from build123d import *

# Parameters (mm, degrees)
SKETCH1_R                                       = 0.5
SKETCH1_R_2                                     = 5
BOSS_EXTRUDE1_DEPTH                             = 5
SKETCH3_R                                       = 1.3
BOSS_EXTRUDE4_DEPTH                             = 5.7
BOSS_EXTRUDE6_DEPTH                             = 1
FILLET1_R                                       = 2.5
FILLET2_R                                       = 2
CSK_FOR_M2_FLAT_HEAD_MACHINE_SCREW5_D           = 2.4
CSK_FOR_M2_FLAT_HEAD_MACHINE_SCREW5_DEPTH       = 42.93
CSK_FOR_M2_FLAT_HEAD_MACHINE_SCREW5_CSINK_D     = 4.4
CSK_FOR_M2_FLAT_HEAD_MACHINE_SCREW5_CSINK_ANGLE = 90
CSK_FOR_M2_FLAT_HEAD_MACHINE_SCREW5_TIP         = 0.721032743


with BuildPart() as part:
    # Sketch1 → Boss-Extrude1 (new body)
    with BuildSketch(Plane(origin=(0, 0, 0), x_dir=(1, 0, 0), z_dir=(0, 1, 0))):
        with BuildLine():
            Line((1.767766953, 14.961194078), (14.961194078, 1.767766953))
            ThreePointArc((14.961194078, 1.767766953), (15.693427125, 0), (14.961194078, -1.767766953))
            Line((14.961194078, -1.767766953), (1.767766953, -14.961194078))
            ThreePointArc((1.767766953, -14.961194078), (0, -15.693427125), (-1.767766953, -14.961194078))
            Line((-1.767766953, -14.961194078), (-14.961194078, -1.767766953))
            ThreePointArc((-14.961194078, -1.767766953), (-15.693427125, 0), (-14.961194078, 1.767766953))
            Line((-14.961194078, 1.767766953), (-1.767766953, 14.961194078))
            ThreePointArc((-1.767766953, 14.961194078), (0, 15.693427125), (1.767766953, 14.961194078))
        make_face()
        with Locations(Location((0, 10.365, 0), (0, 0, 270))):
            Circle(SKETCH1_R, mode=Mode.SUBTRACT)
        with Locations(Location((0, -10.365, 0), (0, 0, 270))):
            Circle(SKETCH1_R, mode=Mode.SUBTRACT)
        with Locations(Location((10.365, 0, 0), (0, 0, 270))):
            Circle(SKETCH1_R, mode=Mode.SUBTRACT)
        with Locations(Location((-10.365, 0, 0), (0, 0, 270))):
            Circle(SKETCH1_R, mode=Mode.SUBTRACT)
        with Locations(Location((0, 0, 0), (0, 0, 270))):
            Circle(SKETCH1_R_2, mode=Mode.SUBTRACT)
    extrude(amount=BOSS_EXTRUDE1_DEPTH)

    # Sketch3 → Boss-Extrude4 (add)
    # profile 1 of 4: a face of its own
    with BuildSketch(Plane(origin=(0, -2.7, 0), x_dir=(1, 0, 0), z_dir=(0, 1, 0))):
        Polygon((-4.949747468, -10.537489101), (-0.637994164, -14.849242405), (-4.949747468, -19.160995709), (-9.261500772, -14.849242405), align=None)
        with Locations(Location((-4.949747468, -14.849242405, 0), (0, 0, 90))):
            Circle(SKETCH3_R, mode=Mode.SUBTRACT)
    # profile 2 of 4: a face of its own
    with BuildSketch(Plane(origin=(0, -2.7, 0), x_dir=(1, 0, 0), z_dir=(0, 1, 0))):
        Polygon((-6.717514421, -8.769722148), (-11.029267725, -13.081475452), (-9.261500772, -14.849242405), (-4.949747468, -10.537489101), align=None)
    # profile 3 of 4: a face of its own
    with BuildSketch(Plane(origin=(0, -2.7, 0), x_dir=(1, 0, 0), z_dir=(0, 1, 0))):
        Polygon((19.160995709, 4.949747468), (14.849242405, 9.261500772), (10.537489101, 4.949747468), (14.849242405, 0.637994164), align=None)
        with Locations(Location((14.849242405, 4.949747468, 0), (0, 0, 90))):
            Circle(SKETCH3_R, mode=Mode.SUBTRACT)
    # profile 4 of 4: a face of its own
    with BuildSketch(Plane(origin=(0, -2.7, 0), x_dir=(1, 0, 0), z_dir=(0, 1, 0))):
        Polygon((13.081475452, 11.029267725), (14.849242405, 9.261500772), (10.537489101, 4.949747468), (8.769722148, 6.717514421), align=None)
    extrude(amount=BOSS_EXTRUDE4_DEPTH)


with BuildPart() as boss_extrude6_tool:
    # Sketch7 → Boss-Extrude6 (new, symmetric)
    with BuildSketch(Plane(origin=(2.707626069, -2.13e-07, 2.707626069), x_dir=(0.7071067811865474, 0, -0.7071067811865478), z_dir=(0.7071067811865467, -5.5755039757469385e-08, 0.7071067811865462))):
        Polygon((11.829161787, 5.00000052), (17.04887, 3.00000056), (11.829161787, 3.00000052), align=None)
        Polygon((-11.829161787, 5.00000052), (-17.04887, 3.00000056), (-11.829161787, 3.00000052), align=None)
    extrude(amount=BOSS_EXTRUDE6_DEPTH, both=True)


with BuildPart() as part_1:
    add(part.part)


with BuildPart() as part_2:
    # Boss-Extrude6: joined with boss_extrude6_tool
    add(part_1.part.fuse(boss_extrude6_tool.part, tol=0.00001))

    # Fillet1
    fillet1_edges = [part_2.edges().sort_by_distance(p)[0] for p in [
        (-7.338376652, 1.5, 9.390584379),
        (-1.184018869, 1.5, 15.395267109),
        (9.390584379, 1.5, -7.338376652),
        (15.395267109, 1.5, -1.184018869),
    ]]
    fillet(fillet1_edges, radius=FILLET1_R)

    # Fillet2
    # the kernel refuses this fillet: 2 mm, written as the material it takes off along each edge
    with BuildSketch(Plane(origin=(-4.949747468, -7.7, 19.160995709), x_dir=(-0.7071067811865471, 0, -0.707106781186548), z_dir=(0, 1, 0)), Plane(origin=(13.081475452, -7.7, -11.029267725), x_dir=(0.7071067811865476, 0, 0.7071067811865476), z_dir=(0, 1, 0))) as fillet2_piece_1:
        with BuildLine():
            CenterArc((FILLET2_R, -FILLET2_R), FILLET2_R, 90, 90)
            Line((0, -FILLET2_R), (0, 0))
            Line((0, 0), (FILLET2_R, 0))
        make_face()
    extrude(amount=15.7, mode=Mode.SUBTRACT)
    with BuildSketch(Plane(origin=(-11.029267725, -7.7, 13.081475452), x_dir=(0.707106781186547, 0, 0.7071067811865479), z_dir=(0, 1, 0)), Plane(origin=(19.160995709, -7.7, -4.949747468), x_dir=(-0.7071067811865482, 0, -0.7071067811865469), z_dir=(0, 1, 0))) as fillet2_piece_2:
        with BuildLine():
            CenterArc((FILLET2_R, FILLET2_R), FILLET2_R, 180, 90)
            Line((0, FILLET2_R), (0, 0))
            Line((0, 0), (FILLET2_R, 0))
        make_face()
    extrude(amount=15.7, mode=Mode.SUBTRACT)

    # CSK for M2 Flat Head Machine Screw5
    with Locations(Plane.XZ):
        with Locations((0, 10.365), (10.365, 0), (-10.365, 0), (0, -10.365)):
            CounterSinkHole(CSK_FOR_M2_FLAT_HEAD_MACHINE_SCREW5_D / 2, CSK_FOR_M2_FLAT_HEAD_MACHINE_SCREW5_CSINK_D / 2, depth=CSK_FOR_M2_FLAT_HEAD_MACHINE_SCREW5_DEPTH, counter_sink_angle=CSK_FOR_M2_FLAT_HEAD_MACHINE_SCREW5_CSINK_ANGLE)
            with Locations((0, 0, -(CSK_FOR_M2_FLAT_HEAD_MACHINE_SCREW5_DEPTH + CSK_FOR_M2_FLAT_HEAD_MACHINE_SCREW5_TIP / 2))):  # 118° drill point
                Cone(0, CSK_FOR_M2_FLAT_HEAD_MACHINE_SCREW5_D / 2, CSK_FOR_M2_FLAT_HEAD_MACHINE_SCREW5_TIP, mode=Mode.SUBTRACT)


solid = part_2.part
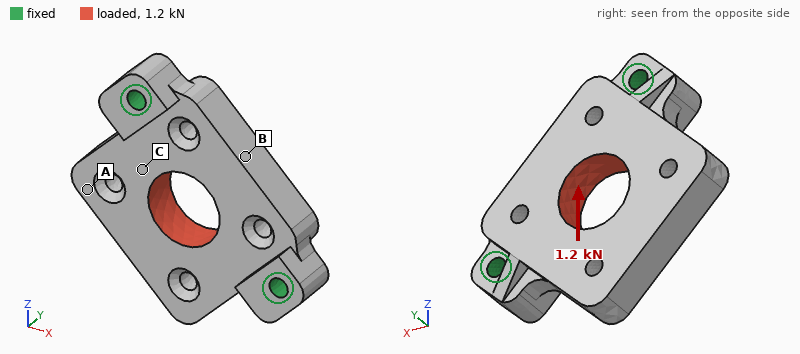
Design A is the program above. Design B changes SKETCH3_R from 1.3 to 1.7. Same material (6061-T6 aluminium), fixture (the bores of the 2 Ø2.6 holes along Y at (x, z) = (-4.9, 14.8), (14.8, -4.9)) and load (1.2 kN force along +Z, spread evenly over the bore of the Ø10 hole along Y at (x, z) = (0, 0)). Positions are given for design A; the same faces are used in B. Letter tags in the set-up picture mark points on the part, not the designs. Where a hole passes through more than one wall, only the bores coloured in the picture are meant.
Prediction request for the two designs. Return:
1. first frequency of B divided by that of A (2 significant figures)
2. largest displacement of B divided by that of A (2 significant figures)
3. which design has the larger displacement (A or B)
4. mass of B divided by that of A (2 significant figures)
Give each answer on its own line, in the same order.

1.0
0.83
A
0.98
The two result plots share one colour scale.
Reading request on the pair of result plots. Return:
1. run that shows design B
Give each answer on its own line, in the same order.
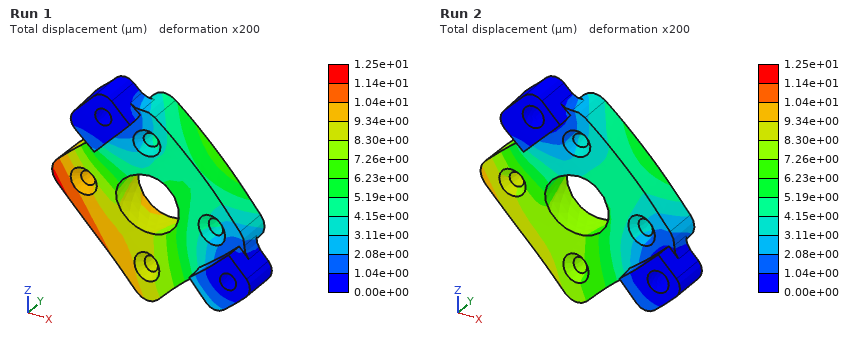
Run 2
